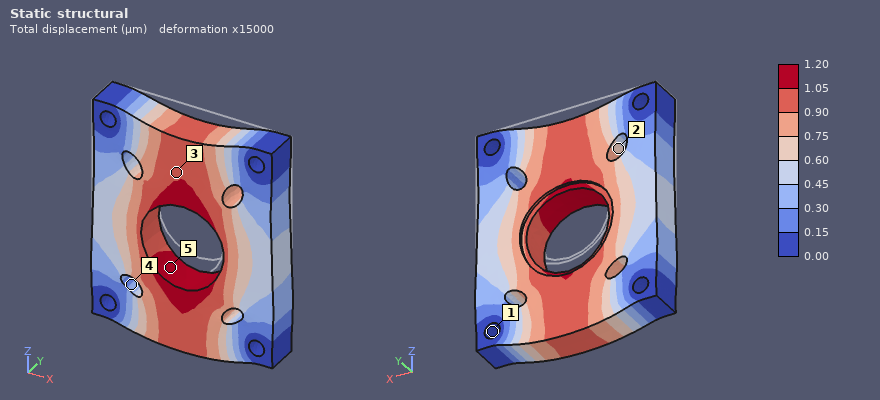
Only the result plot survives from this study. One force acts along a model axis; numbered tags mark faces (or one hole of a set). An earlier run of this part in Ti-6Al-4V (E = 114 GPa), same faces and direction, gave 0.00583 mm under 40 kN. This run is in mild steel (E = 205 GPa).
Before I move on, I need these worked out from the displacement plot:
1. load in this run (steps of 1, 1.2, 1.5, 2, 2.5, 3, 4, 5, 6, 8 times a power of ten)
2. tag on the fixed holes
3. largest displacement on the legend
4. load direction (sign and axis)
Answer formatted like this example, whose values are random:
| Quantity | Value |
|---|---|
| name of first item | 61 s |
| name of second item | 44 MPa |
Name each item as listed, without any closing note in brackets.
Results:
| Quantity | Value |
|---|---|
| load in this run | 15 kN |
| tag on the fixed holes | 1 |
| largest displacement on the legend | 1.20 µm |
| load direction | -Z |
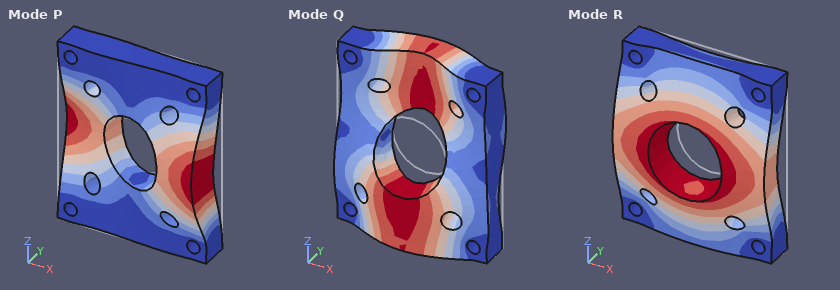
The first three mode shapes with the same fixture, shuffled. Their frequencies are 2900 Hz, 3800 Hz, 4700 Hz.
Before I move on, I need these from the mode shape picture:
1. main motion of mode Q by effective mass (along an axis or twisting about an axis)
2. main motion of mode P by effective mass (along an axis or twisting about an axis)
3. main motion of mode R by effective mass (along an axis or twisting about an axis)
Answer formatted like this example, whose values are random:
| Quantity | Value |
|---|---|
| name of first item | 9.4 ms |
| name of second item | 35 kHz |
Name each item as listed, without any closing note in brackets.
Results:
| Quantity | Value |
|---|---|
| main motion of mode Q by effective mass | twisting about X |
| main motion of mode P by effective mass | twisting about Z |
| main motion of mode R by effective mass | along Y |
